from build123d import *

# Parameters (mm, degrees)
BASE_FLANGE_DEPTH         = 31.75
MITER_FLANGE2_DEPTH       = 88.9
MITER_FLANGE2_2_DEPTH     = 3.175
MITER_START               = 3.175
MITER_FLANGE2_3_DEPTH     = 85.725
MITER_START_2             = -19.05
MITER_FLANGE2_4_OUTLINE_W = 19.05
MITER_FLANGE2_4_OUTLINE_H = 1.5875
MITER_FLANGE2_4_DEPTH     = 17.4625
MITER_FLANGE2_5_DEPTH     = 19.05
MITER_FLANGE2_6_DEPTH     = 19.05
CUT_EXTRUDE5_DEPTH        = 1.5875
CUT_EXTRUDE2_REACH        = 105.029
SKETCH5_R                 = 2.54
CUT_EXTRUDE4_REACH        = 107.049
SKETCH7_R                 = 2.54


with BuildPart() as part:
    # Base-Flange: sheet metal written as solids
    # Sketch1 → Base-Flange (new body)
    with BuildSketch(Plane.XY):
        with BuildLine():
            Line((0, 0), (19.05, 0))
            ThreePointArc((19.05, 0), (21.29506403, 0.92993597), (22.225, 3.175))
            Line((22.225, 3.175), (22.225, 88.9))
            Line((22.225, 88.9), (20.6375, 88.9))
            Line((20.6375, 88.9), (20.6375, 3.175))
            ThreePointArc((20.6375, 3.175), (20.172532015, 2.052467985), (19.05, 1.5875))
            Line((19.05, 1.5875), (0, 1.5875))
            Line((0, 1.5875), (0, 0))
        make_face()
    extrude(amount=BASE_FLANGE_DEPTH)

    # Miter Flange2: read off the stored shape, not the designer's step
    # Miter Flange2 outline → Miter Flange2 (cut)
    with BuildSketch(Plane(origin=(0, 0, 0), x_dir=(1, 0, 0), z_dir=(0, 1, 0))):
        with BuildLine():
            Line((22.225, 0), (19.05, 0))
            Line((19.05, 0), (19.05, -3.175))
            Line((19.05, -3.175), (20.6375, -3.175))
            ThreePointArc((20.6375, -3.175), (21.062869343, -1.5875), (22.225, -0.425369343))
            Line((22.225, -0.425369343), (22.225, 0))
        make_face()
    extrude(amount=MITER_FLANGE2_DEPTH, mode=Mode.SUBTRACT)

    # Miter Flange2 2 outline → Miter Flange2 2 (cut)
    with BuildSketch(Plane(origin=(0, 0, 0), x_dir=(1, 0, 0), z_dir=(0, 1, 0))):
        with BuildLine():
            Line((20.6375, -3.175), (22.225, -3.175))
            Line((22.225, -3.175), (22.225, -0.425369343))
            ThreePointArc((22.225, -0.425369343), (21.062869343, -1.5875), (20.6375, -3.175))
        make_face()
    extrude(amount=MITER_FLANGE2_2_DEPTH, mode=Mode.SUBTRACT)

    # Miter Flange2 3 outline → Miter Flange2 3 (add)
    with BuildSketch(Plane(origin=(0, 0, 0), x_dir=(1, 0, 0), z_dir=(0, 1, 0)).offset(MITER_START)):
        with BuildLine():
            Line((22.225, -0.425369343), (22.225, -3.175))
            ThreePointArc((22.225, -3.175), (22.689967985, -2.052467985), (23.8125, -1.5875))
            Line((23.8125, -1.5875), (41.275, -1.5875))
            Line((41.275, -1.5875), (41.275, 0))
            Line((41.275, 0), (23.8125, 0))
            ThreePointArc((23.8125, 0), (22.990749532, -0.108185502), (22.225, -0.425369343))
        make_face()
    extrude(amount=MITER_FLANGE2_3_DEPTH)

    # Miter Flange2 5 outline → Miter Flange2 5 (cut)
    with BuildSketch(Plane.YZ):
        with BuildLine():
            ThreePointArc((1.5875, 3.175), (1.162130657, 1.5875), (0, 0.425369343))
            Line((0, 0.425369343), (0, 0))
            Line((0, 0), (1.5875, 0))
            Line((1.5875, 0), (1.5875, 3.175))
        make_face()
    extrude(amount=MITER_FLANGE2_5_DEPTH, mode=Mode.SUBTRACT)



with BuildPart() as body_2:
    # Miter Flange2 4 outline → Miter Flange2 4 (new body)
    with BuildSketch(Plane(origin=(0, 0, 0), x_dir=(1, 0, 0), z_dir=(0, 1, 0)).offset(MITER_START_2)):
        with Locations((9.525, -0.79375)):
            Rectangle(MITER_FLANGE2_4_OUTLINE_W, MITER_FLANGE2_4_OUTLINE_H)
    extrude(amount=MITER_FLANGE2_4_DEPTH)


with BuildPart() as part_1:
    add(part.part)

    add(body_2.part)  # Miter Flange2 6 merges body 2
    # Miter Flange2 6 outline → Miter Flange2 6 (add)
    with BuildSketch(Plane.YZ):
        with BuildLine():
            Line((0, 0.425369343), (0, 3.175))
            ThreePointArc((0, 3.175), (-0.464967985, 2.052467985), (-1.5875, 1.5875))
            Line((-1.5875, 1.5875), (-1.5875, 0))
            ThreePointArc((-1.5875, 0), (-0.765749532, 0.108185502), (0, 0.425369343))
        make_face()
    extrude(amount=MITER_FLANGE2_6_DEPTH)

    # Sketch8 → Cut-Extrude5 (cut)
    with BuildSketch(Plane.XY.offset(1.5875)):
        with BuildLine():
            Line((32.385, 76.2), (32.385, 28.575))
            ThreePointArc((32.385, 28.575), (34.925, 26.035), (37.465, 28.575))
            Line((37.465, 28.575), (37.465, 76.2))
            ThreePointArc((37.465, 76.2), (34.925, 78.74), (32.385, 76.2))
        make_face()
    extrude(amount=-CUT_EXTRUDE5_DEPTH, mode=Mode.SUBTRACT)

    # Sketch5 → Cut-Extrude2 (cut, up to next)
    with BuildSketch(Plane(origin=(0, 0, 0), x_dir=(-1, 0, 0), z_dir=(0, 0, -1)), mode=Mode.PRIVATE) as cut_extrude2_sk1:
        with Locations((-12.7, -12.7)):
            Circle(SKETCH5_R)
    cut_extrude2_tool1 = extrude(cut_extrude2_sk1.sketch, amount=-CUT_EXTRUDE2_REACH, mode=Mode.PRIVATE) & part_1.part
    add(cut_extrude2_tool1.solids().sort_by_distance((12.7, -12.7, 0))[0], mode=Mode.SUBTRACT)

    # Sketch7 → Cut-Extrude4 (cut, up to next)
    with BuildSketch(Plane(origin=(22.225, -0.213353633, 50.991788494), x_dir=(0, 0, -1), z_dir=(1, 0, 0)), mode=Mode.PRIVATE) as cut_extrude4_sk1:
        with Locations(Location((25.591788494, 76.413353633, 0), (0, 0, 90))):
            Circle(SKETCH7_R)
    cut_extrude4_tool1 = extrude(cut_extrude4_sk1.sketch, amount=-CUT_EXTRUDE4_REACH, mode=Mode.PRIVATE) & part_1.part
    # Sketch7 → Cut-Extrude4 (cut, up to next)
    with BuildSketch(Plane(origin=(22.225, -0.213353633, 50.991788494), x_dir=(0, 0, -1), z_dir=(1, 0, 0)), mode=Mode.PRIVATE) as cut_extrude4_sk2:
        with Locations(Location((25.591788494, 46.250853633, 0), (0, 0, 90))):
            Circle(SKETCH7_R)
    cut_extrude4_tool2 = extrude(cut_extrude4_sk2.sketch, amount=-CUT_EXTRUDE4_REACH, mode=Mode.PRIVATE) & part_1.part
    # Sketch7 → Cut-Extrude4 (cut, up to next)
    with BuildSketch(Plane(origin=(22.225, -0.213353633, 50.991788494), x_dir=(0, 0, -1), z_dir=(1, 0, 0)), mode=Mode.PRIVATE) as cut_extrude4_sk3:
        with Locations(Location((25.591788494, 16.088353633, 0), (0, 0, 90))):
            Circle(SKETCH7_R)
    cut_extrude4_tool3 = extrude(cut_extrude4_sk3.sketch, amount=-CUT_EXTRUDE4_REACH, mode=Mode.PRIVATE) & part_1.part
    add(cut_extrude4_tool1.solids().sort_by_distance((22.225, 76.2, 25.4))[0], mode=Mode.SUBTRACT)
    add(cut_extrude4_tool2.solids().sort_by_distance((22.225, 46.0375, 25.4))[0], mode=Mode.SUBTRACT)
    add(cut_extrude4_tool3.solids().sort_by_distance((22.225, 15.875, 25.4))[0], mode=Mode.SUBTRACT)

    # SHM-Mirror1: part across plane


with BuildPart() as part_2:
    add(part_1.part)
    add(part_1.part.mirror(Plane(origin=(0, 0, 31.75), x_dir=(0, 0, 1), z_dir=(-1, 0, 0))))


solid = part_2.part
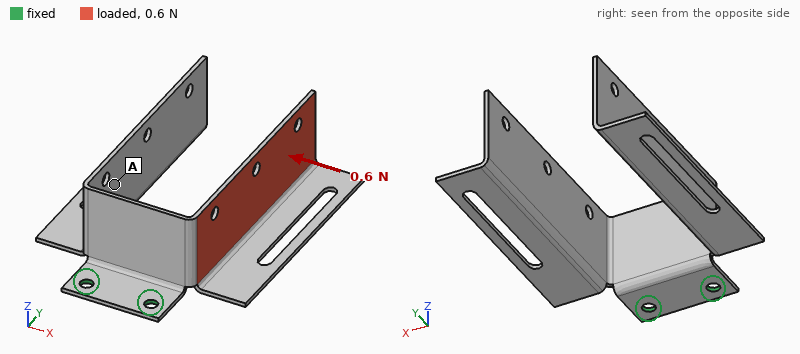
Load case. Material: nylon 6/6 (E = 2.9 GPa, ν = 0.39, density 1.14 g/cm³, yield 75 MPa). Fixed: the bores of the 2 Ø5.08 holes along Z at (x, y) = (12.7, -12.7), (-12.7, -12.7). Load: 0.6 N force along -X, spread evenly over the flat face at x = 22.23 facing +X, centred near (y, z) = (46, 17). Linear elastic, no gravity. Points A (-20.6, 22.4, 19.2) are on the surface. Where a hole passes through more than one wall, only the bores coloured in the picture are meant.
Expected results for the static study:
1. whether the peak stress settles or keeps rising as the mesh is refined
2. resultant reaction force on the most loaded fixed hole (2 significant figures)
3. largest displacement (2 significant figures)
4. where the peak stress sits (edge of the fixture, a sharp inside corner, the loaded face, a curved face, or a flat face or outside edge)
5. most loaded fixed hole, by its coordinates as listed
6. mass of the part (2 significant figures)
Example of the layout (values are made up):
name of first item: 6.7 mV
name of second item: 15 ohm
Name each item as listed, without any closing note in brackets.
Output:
whether the peak stress settles or keeps rising as the mesh is refined: keeps rising
resultant reaction force on the most loaded fixed hole: 1.5 N
largest displacement: 1.7 mm
where the peak stress sits: a sharp inside corner
most loaded fixed hole, by its coordinates as listed: (-12.7, -12.7)
mass of the part: 18 g
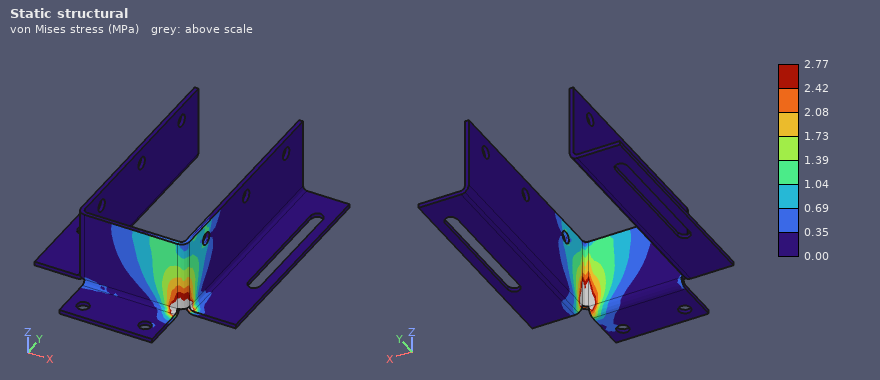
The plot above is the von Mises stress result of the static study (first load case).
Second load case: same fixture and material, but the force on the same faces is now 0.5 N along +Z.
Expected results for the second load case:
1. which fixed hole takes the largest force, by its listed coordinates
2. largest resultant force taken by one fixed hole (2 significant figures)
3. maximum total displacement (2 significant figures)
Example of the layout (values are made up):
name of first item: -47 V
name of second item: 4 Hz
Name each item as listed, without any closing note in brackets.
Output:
which fixed hole takes the largest force, by its listed coordinates: (12.7, -12.7)
largest resultant force taken by one fixed hole: 0.74 N
maximum total displacement: 1.6 mm
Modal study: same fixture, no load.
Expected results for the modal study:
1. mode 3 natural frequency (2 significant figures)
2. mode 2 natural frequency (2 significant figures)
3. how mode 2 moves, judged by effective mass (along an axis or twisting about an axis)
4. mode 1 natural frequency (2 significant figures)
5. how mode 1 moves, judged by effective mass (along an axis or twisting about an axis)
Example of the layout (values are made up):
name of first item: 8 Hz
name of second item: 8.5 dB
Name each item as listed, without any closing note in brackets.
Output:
mode 3 natural frequency: 45 Hz
mode 2 natural frequency: 40 Hz
how mode 2 moves, judged by effective mass: along X
mode 1 natural frequency: 33 Hz
how mode 1 moves, judged by effective mass: along Z
